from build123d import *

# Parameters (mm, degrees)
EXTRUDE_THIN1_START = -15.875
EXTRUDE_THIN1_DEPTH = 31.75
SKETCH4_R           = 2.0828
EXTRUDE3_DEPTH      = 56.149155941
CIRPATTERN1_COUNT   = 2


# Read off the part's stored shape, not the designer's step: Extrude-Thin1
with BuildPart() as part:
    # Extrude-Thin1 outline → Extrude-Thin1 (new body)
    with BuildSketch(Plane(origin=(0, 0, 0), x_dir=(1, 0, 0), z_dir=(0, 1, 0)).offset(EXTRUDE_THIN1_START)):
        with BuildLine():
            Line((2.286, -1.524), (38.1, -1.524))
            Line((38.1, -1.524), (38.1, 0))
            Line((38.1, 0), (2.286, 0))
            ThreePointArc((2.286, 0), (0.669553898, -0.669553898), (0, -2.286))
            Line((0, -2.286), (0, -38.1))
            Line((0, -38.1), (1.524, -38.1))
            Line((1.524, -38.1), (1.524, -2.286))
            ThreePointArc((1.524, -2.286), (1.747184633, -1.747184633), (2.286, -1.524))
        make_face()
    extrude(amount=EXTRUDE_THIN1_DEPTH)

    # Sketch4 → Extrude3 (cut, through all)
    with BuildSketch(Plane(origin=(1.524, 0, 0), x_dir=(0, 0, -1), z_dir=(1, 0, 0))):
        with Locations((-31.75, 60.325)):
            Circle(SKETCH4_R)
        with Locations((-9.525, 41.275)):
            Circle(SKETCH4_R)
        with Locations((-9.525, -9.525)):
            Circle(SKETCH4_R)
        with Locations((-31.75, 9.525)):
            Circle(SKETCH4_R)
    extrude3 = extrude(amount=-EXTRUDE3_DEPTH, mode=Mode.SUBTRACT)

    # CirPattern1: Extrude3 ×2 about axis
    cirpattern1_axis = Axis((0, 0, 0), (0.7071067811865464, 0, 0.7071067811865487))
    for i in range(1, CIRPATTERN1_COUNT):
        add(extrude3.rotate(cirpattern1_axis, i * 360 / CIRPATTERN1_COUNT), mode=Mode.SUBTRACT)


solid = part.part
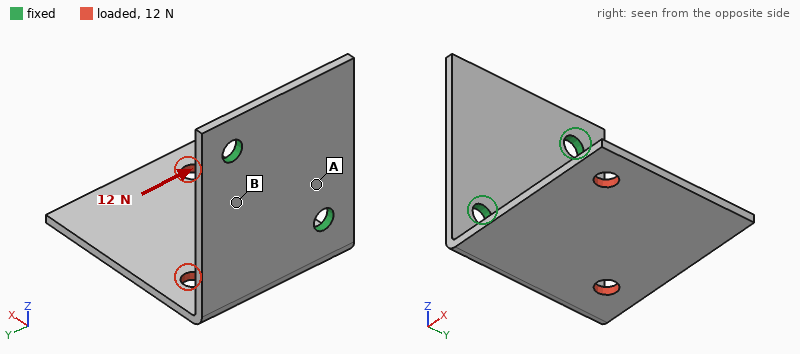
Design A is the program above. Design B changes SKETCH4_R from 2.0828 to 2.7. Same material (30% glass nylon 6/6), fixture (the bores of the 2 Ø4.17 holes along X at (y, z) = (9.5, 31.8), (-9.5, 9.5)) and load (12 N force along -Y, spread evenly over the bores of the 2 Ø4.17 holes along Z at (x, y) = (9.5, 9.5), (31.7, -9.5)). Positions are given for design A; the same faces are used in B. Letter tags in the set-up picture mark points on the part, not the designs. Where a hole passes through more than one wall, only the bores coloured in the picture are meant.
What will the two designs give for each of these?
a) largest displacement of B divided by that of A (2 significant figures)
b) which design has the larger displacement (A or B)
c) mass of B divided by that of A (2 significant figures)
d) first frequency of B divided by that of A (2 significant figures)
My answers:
0.86
A
0.98
1.0
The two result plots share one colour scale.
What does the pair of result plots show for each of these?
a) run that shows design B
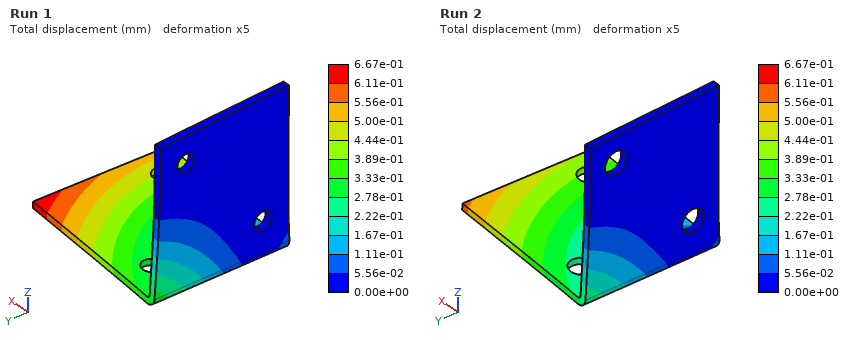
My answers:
Run 2
